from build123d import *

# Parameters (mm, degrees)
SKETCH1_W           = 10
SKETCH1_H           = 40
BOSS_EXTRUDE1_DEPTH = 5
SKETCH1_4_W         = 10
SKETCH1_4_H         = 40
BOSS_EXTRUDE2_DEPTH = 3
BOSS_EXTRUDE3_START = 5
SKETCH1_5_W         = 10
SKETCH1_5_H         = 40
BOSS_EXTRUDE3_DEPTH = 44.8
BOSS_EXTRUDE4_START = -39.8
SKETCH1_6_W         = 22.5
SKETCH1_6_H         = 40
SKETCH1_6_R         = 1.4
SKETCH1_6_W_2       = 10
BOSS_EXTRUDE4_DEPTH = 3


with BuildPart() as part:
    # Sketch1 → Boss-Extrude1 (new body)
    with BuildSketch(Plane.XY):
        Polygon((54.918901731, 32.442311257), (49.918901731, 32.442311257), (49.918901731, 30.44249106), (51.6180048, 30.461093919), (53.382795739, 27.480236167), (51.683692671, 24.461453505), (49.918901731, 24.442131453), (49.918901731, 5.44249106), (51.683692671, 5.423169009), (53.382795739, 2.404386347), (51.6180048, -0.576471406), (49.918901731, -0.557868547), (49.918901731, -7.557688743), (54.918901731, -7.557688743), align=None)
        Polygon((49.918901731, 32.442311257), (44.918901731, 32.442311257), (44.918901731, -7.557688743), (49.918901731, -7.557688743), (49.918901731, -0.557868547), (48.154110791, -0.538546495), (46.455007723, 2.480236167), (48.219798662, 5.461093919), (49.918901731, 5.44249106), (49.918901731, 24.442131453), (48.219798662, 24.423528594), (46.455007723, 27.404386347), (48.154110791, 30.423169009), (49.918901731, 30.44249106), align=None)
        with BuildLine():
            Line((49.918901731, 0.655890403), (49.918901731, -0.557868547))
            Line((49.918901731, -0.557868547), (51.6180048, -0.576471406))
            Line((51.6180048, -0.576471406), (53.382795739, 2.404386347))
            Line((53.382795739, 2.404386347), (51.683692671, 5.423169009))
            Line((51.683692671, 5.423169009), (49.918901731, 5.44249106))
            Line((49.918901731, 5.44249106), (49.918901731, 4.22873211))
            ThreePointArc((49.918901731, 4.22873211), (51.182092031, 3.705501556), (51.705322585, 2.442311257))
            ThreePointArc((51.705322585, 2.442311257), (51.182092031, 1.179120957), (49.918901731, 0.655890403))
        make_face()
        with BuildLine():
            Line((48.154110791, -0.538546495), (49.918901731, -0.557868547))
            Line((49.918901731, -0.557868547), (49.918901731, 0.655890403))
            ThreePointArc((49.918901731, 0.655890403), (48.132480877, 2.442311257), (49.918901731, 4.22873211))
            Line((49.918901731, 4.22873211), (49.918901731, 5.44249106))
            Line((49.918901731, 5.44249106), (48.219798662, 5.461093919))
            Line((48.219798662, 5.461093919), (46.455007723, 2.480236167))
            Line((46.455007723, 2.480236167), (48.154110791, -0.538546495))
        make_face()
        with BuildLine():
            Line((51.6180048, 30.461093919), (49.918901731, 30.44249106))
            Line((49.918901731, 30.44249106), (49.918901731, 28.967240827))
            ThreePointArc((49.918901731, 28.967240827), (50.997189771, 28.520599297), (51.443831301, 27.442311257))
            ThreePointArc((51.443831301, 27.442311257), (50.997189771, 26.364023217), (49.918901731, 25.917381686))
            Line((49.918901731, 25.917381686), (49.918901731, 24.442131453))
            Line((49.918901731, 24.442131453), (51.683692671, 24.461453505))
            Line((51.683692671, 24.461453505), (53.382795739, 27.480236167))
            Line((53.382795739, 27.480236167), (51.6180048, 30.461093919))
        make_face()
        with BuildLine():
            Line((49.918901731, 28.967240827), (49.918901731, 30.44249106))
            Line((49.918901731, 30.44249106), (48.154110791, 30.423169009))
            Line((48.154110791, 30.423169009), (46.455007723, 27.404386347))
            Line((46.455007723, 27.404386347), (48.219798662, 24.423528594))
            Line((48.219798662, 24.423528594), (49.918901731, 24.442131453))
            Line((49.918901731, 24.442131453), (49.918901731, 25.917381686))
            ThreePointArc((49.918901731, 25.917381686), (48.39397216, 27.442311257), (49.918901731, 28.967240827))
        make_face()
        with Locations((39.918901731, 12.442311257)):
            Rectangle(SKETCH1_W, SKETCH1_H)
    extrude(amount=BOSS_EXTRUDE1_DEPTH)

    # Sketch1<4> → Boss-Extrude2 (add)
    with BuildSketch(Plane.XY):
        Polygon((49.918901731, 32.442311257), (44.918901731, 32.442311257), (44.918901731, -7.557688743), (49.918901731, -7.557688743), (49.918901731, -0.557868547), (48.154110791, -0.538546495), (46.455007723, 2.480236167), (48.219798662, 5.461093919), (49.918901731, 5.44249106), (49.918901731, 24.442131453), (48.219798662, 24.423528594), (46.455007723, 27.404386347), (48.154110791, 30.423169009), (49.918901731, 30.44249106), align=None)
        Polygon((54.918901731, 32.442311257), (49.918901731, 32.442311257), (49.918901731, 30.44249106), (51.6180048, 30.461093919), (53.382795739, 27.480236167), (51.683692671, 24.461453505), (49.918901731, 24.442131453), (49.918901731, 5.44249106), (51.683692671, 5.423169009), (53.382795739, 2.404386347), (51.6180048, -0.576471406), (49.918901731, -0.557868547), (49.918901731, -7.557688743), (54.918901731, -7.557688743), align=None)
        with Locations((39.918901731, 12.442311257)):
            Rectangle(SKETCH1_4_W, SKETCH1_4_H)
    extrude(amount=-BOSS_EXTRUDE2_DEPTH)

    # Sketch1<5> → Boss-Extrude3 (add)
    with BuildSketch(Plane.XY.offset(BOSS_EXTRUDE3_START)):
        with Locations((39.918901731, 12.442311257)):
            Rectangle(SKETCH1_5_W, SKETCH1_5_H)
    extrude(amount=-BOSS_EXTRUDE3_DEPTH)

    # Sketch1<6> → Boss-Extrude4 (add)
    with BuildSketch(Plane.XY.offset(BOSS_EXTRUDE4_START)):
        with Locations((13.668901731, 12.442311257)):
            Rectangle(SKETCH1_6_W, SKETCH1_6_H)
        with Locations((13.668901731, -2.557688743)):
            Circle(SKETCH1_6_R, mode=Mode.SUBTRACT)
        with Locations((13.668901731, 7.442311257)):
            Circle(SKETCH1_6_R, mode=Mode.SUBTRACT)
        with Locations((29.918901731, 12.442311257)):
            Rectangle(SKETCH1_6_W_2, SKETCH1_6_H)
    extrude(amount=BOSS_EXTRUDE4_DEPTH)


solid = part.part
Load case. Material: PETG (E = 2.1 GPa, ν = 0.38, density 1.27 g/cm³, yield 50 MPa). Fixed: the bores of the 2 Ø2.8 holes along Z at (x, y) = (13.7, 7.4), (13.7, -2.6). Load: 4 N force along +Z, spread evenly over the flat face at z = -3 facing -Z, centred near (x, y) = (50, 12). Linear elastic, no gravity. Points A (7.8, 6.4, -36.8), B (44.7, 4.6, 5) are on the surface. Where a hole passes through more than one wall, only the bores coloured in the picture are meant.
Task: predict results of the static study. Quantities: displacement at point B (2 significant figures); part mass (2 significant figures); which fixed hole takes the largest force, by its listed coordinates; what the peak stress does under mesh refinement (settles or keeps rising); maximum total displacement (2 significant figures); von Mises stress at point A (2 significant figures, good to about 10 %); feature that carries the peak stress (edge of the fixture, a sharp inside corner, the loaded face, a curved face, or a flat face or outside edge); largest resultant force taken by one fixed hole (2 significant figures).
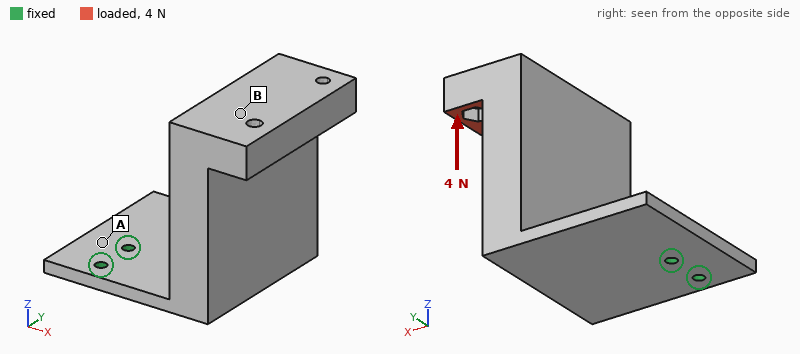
0.67 mm
31 g
(13.7, 7.4)
keeps rising
0.78 mm
0.86 MPa
edge of the fixture
4.2 N
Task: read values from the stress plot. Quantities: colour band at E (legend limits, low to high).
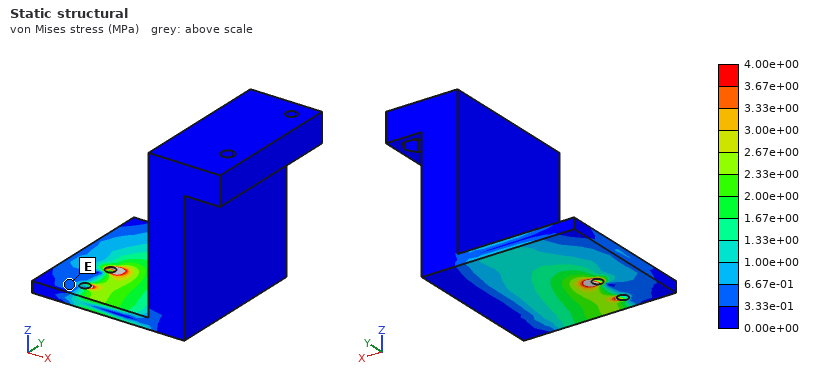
3.33e-01 to 6.67e-01 MPa
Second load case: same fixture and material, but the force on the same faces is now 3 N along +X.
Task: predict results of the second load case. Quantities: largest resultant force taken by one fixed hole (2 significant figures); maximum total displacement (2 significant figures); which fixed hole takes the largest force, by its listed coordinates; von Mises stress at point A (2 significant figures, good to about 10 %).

3.9 N
0.74 mm
(13.7, 7.4)
0.77 MPa
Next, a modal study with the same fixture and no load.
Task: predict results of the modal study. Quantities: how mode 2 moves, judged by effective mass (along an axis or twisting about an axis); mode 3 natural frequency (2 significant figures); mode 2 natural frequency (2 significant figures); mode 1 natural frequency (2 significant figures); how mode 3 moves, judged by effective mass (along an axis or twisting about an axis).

along Y
440 Hz
140 Hz
82 Hz
along Z
